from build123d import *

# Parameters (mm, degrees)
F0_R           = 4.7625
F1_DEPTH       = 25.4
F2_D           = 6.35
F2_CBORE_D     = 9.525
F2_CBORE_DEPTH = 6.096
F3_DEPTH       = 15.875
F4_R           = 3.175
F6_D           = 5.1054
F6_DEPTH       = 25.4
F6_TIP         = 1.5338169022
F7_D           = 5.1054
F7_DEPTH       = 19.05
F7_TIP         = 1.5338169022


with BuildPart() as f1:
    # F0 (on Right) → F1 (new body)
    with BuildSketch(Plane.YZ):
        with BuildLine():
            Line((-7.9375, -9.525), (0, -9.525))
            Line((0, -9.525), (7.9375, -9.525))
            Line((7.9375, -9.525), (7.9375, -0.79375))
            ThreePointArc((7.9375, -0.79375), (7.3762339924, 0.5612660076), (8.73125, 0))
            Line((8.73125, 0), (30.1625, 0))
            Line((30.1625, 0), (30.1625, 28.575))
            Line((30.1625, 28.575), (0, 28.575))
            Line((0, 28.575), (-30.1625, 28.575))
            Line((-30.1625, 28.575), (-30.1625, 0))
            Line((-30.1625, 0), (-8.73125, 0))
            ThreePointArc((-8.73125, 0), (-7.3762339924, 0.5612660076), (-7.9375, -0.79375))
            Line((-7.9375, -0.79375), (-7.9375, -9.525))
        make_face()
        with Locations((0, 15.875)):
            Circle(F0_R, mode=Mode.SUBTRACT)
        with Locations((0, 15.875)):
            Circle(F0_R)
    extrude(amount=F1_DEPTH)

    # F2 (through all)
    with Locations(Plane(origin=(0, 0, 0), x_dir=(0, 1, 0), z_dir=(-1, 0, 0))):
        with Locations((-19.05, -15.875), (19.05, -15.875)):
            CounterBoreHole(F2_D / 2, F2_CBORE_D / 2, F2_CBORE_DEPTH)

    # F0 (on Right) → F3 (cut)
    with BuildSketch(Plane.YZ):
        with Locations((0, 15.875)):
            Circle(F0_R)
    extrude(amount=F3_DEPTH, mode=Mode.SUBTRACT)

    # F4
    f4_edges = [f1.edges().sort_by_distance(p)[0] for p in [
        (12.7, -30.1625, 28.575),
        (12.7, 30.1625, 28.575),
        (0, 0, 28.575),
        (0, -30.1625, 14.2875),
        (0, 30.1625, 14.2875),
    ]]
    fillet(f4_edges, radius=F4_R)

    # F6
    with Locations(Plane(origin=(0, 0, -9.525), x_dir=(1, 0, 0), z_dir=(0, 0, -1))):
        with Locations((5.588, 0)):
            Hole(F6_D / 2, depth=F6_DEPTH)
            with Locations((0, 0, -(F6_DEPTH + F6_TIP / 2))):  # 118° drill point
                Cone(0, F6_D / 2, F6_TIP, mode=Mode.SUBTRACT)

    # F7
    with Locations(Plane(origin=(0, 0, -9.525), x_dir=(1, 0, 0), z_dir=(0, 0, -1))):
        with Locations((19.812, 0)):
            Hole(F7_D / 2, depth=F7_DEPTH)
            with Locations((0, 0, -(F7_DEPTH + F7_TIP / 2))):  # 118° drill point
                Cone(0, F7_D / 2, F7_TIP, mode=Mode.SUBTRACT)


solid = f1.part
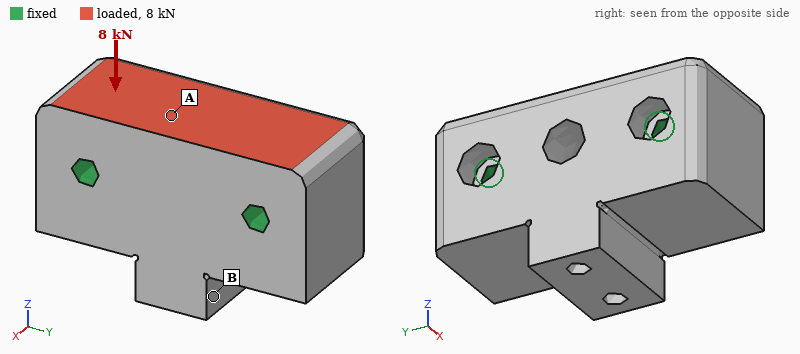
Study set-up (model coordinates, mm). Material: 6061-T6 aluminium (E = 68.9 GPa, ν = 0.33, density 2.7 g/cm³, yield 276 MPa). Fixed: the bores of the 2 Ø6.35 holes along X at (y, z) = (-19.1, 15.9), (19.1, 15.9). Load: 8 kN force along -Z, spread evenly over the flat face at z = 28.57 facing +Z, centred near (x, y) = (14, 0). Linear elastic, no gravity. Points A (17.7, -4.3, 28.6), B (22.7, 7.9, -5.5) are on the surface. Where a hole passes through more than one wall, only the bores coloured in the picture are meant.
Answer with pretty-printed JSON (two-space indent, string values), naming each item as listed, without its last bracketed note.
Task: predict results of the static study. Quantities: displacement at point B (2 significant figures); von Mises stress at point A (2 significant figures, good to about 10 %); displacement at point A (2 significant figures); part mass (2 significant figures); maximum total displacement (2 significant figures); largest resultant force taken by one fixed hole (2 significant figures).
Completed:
{
  "displacement at point B": "1.6 µm",
  "von Mises stress at point A": "7.2 MPa",
  "displacement at point A": "3.0 µm",
  "part mass": "120 g",
  "maximum total displacement": "3.6 µm",
  "largest resultant force taken by one fixed hole": "4.0 kN"
}
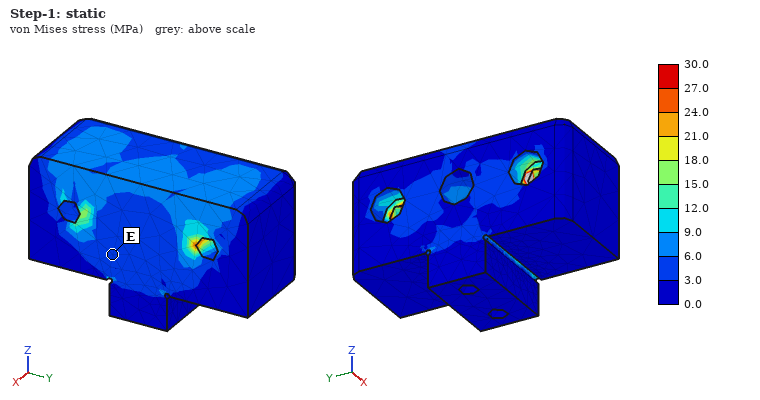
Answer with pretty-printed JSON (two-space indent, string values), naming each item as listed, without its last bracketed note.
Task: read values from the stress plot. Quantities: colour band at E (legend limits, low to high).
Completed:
{
  "colour band at E": "3.0 to 6.0 MPa"
}
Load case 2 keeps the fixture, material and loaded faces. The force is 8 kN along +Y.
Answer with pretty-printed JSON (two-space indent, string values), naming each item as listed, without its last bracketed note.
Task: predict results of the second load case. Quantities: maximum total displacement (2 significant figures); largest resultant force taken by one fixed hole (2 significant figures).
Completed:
{
  "maximum total displacement": "5.1 µm",
  "largest resultant force taken by one fixed hole": "4.5 kN"
}
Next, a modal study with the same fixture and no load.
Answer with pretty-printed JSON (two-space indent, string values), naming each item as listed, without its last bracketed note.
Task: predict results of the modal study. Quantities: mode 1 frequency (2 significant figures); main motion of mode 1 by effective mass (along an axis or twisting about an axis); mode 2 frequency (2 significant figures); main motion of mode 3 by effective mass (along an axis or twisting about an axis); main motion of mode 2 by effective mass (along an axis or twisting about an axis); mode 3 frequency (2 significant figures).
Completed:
{
  "mode 1 frequency": "18 kHz",
  "main motion of mode 1 by effective mass": "along X",
  "mode 2 frequency": "27 kHz",
  "main motion of mode 3 by effective mass": "along Y",
  "main motion of mode 2 by effective mass": "along Z",
  "mode 3 frequency": "29 kHz"
}
